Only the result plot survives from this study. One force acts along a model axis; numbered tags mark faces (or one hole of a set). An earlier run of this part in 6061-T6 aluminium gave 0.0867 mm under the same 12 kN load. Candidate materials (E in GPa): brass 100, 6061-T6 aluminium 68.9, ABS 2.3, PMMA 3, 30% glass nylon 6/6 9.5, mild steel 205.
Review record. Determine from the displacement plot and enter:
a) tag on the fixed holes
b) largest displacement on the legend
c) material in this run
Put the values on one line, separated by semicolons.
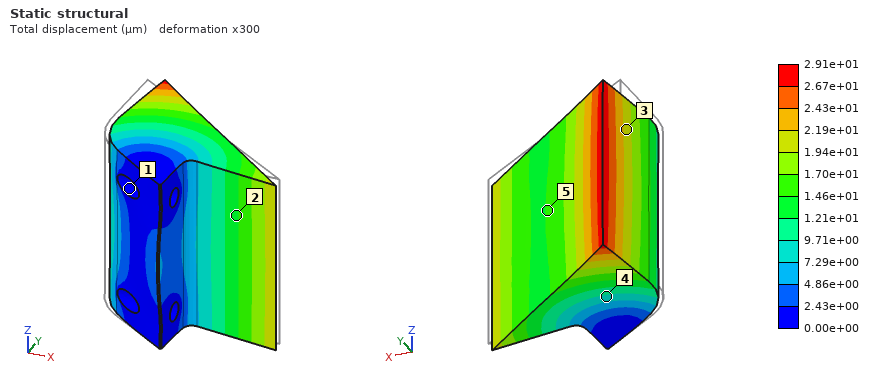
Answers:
1; 2.91e+01 µm; mild steel
